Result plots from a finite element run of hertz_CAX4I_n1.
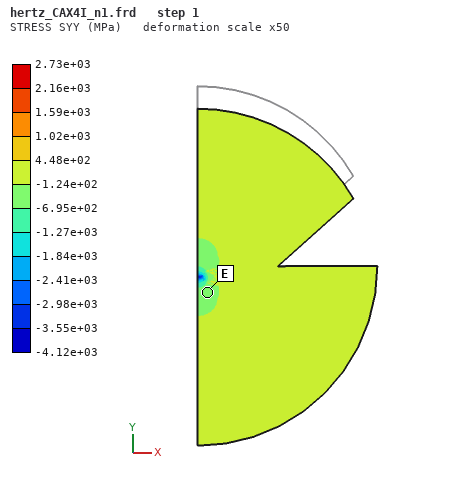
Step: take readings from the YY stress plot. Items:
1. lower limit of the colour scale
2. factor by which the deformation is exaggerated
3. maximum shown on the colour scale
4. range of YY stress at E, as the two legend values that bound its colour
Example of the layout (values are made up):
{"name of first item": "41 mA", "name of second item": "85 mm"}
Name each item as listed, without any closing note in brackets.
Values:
{"lower limit of the colour scale": "-4.12e+03 MPa", "factor by which the deformation is exaggerated": "50", "maximum shown on the colour scale": "2.73e+03 MPa", "range of YY stress at E, as the two legend values that bound its colour": "-6.95e+02 to -1.24e+02 MPa"}
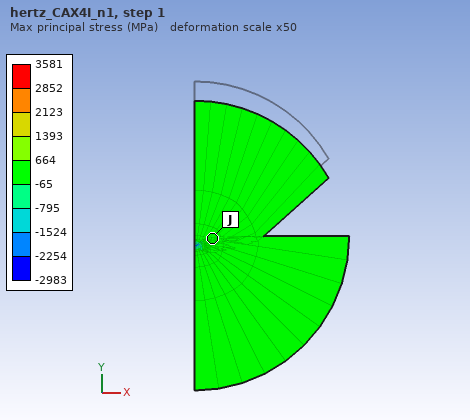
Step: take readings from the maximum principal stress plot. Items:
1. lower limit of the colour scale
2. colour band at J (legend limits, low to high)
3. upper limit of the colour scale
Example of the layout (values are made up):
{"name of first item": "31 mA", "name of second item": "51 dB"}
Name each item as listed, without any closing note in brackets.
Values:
{"lower limit of the colour scale": "-2983 MPa", "colour band at J": "-65 to 664 MPa", "upper limit of the colour scale": "3581 MPa"}
